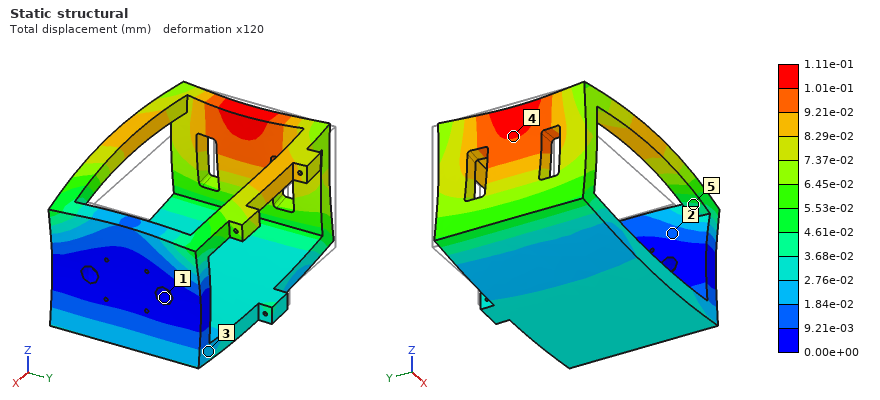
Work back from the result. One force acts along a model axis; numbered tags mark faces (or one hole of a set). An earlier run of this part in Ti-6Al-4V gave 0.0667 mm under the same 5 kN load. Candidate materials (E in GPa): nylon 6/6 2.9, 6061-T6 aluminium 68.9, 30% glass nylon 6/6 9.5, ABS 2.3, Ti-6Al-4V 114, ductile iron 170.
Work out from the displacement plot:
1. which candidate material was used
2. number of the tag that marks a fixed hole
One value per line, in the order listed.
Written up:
6061-T6 aluminium
1
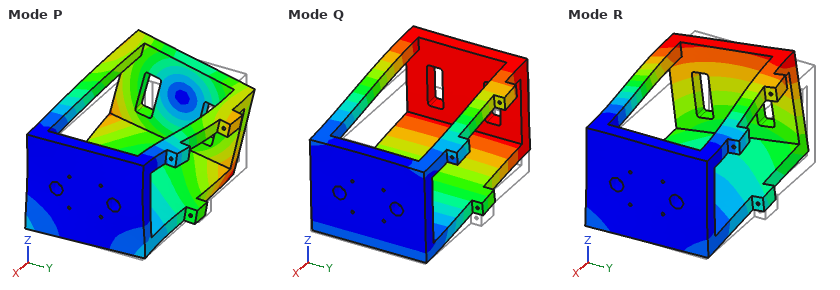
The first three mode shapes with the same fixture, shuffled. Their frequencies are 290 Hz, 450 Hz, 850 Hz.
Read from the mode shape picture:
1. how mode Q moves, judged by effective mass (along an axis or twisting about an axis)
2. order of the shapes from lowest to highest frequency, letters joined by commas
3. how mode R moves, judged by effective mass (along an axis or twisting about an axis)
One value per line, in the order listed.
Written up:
along Z
Q, R, P
along Y
